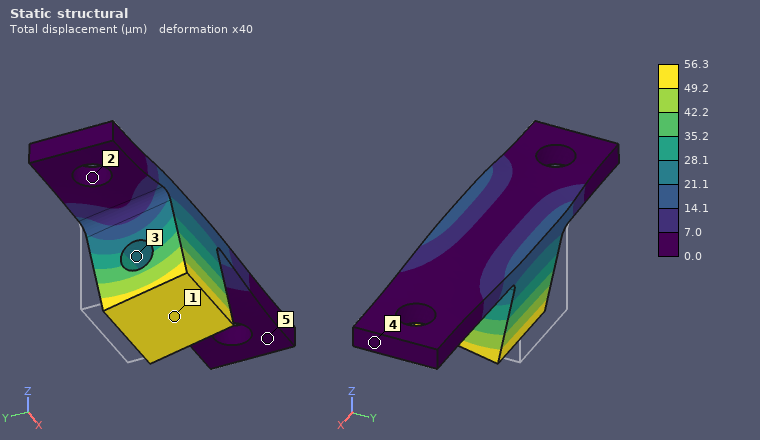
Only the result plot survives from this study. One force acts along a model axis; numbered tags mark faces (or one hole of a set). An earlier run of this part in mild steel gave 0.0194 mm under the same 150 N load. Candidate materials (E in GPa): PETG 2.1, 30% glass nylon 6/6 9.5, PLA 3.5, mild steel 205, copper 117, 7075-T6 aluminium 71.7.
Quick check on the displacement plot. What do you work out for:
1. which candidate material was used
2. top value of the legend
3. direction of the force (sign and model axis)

7075-T6 aluminium
56.3 µm
-Y
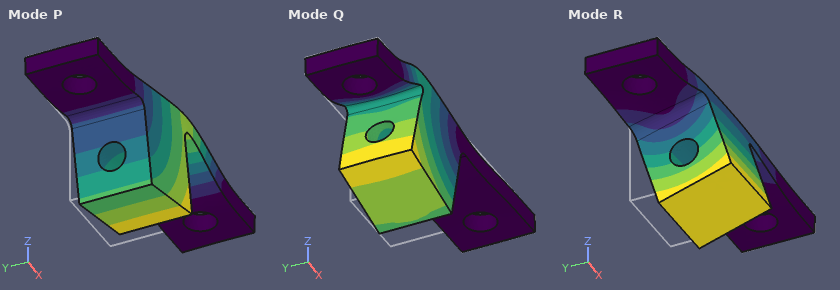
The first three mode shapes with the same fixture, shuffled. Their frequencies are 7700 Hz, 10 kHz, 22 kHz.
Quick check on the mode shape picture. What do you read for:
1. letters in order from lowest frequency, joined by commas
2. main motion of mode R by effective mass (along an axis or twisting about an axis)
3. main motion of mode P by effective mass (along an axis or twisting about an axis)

R, P, Q
along Y
along Z
